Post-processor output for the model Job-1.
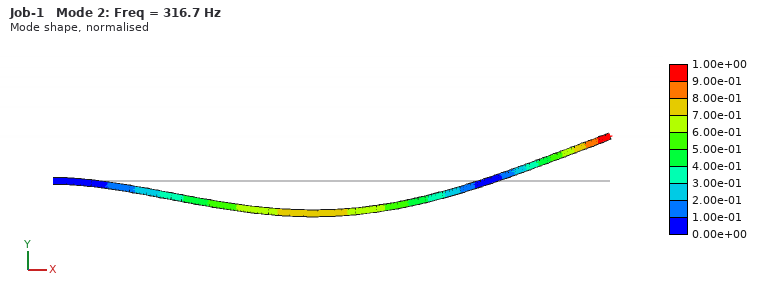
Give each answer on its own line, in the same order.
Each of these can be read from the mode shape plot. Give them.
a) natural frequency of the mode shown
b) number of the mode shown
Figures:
316.7 Hz
2
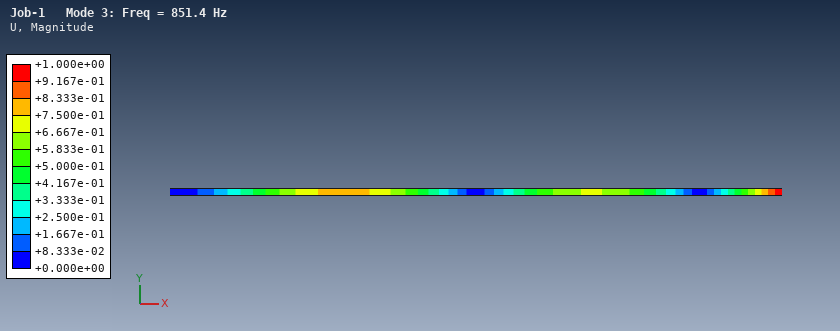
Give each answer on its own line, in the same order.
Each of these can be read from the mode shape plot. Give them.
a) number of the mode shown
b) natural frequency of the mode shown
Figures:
3
851.4 Hz
